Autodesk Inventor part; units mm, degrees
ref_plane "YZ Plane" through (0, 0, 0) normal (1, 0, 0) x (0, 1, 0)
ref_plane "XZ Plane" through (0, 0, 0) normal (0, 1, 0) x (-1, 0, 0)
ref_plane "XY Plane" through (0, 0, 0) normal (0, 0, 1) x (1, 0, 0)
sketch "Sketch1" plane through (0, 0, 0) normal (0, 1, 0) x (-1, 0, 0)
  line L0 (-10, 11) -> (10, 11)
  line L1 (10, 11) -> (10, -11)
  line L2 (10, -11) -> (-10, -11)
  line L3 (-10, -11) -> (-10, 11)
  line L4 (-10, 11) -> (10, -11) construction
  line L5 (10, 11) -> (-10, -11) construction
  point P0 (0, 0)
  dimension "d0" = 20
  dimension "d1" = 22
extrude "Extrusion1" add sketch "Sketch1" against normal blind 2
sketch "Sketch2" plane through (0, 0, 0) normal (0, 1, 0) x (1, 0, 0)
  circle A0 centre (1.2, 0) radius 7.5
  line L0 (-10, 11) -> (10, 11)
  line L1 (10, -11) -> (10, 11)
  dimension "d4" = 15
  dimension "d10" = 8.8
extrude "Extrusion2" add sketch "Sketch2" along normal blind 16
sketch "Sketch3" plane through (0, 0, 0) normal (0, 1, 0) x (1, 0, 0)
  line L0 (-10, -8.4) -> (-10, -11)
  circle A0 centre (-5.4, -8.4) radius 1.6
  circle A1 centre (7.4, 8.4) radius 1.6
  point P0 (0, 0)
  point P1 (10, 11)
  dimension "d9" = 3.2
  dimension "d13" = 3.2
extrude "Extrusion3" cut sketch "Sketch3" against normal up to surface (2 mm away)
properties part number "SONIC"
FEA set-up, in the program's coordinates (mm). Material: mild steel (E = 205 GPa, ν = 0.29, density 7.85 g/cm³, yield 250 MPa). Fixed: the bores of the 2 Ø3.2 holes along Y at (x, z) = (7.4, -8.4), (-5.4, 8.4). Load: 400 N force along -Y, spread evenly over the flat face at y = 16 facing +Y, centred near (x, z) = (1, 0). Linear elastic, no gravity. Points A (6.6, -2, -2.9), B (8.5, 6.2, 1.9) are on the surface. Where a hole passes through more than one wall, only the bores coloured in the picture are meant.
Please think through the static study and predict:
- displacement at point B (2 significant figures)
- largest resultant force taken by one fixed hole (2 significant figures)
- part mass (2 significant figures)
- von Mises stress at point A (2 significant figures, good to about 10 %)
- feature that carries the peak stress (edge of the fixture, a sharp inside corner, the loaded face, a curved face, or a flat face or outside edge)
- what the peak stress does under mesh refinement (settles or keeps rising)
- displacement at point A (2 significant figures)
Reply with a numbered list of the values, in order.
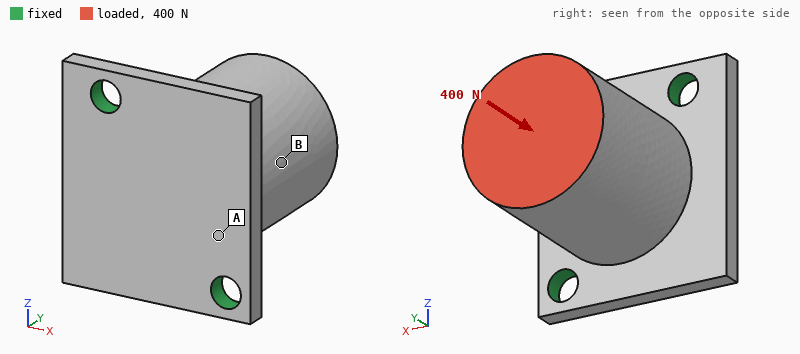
1. 1.7 µm
2. 220 N
3. 29 g
4. 14 MPa
5. edge of the fixture
6. keeps rising
7. 1.3 µm
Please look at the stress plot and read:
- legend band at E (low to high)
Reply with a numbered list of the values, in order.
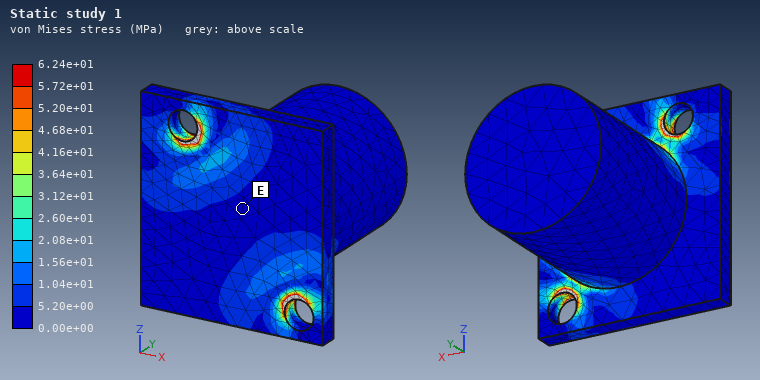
1. 0.00e+00 to 5.20e+00 MPa
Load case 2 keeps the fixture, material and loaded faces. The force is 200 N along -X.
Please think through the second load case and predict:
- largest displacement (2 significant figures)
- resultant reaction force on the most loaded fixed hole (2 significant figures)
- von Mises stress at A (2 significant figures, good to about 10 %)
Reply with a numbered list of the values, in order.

1. 30 µm
2. 160 N
3. 52 MPa
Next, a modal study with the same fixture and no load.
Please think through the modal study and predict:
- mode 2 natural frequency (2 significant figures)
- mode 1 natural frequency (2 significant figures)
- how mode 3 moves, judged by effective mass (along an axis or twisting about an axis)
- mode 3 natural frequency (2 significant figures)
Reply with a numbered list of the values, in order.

1. 14 kHz
2. 3900 Hz
3. along Y
4. 16 kHz
